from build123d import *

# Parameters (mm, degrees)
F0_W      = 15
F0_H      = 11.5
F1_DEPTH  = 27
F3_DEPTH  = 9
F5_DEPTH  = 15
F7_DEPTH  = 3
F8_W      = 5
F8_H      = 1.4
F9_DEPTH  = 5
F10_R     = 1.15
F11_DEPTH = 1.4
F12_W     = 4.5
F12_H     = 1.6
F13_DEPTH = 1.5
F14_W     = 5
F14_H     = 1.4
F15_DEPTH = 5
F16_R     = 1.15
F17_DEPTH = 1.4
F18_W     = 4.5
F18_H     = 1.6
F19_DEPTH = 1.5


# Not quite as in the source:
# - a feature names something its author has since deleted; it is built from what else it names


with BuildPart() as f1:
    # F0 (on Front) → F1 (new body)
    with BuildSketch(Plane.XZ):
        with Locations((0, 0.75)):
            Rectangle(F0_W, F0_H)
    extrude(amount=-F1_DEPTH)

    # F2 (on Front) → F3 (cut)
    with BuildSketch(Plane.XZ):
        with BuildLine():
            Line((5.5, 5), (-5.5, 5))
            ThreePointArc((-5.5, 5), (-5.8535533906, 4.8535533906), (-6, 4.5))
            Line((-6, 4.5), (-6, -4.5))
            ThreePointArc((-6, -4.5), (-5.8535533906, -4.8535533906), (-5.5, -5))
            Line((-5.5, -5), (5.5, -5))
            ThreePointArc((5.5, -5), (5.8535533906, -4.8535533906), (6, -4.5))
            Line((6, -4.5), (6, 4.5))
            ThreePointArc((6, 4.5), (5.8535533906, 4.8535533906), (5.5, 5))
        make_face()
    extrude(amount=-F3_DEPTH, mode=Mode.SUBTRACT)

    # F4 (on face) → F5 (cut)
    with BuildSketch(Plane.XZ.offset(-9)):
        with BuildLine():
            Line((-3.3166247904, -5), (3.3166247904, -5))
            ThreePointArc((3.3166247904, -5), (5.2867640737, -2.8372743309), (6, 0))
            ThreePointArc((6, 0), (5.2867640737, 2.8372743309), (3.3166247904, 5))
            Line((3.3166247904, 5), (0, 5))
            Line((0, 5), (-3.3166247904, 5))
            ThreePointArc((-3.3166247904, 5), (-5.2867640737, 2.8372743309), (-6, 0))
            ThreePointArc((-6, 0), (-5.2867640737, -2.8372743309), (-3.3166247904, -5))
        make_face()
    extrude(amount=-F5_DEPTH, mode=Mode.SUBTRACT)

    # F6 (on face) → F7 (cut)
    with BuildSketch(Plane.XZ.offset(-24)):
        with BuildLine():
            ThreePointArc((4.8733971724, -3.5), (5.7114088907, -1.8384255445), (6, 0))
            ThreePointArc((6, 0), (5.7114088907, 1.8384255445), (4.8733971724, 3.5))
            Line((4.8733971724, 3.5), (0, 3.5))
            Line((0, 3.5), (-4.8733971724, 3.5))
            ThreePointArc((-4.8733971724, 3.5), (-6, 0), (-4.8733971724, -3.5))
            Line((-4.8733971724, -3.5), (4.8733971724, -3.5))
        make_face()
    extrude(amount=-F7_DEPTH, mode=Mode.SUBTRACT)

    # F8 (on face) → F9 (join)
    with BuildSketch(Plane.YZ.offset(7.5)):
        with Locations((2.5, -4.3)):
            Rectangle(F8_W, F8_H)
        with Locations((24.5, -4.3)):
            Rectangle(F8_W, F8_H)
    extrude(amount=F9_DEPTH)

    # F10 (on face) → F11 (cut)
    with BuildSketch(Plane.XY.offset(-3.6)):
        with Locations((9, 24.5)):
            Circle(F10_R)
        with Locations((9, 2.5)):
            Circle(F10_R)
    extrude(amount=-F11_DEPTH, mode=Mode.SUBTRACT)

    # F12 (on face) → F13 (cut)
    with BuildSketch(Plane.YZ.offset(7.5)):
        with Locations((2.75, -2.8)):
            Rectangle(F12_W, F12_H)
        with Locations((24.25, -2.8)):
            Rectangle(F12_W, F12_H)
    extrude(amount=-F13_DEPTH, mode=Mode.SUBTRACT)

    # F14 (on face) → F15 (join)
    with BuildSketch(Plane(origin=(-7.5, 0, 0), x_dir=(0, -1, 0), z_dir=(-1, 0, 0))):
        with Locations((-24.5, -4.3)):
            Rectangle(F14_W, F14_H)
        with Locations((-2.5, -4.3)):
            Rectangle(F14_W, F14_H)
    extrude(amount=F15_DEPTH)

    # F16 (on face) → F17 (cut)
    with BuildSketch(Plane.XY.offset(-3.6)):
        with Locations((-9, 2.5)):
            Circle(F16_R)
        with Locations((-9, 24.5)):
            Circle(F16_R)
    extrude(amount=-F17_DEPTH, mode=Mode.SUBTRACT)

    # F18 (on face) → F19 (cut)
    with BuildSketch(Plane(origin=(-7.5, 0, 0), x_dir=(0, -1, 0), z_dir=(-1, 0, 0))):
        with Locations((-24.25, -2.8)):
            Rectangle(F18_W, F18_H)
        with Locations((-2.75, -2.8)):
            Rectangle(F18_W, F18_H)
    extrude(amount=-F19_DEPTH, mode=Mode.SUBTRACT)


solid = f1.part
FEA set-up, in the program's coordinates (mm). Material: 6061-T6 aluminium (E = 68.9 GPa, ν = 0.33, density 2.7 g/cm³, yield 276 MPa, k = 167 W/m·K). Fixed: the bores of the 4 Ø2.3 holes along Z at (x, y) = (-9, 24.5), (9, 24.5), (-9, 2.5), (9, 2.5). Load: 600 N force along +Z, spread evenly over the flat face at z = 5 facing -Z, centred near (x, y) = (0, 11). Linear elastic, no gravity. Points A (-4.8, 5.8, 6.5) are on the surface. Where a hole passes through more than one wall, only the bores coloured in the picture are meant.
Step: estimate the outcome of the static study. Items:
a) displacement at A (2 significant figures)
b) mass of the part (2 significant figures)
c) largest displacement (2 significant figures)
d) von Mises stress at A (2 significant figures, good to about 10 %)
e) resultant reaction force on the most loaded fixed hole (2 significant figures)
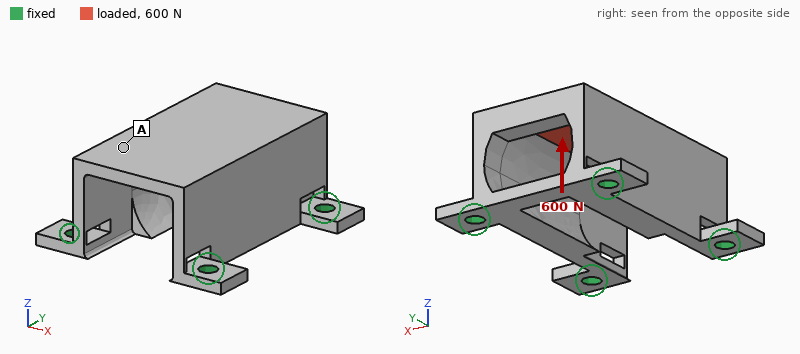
19 µm
5.0 g
39 µm
22 MPa
200 N
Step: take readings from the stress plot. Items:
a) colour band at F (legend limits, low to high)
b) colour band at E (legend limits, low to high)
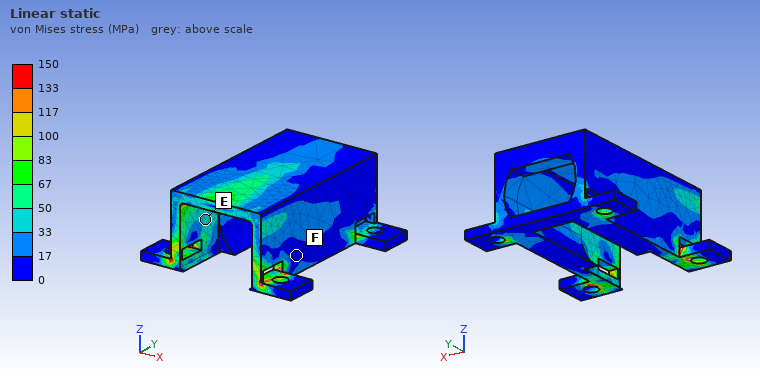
0 to 17 MPa
33 to 50 MPa
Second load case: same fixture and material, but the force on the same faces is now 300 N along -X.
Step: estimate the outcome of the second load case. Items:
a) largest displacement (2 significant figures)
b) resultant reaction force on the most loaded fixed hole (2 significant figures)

57 µm
210 N
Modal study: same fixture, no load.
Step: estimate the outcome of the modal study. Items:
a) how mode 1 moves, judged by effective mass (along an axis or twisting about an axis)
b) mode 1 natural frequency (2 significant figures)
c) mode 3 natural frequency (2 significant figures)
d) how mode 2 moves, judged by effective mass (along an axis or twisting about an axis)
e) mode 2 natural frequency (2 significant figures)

along X
8000 Hz
18 kHz
twisting about Z
17 kHz
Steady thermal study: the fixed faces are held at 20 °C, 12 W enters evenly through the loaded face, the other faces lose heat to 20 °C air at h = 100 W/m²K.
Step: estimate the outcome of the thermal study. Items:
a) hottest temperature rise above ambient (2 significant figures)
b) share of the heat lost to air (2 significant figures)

22 K
22 %
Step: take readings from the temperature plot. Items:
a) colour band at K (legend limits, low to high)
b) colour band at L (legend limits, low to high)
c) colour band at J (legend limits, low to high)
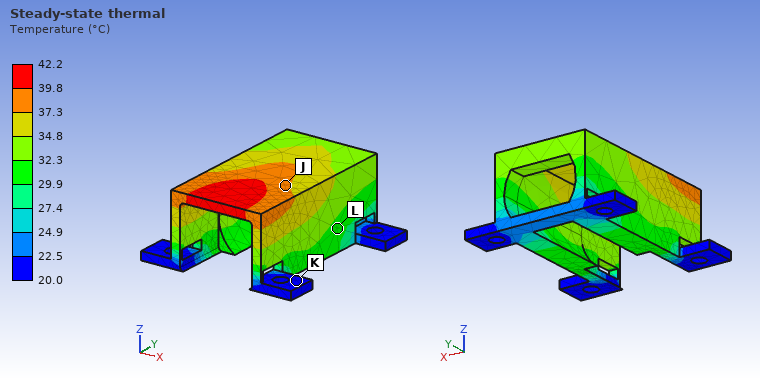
20.0 to 22.5 °C
29.9 to 32.3 °C
37.3 to 39.8 °C
